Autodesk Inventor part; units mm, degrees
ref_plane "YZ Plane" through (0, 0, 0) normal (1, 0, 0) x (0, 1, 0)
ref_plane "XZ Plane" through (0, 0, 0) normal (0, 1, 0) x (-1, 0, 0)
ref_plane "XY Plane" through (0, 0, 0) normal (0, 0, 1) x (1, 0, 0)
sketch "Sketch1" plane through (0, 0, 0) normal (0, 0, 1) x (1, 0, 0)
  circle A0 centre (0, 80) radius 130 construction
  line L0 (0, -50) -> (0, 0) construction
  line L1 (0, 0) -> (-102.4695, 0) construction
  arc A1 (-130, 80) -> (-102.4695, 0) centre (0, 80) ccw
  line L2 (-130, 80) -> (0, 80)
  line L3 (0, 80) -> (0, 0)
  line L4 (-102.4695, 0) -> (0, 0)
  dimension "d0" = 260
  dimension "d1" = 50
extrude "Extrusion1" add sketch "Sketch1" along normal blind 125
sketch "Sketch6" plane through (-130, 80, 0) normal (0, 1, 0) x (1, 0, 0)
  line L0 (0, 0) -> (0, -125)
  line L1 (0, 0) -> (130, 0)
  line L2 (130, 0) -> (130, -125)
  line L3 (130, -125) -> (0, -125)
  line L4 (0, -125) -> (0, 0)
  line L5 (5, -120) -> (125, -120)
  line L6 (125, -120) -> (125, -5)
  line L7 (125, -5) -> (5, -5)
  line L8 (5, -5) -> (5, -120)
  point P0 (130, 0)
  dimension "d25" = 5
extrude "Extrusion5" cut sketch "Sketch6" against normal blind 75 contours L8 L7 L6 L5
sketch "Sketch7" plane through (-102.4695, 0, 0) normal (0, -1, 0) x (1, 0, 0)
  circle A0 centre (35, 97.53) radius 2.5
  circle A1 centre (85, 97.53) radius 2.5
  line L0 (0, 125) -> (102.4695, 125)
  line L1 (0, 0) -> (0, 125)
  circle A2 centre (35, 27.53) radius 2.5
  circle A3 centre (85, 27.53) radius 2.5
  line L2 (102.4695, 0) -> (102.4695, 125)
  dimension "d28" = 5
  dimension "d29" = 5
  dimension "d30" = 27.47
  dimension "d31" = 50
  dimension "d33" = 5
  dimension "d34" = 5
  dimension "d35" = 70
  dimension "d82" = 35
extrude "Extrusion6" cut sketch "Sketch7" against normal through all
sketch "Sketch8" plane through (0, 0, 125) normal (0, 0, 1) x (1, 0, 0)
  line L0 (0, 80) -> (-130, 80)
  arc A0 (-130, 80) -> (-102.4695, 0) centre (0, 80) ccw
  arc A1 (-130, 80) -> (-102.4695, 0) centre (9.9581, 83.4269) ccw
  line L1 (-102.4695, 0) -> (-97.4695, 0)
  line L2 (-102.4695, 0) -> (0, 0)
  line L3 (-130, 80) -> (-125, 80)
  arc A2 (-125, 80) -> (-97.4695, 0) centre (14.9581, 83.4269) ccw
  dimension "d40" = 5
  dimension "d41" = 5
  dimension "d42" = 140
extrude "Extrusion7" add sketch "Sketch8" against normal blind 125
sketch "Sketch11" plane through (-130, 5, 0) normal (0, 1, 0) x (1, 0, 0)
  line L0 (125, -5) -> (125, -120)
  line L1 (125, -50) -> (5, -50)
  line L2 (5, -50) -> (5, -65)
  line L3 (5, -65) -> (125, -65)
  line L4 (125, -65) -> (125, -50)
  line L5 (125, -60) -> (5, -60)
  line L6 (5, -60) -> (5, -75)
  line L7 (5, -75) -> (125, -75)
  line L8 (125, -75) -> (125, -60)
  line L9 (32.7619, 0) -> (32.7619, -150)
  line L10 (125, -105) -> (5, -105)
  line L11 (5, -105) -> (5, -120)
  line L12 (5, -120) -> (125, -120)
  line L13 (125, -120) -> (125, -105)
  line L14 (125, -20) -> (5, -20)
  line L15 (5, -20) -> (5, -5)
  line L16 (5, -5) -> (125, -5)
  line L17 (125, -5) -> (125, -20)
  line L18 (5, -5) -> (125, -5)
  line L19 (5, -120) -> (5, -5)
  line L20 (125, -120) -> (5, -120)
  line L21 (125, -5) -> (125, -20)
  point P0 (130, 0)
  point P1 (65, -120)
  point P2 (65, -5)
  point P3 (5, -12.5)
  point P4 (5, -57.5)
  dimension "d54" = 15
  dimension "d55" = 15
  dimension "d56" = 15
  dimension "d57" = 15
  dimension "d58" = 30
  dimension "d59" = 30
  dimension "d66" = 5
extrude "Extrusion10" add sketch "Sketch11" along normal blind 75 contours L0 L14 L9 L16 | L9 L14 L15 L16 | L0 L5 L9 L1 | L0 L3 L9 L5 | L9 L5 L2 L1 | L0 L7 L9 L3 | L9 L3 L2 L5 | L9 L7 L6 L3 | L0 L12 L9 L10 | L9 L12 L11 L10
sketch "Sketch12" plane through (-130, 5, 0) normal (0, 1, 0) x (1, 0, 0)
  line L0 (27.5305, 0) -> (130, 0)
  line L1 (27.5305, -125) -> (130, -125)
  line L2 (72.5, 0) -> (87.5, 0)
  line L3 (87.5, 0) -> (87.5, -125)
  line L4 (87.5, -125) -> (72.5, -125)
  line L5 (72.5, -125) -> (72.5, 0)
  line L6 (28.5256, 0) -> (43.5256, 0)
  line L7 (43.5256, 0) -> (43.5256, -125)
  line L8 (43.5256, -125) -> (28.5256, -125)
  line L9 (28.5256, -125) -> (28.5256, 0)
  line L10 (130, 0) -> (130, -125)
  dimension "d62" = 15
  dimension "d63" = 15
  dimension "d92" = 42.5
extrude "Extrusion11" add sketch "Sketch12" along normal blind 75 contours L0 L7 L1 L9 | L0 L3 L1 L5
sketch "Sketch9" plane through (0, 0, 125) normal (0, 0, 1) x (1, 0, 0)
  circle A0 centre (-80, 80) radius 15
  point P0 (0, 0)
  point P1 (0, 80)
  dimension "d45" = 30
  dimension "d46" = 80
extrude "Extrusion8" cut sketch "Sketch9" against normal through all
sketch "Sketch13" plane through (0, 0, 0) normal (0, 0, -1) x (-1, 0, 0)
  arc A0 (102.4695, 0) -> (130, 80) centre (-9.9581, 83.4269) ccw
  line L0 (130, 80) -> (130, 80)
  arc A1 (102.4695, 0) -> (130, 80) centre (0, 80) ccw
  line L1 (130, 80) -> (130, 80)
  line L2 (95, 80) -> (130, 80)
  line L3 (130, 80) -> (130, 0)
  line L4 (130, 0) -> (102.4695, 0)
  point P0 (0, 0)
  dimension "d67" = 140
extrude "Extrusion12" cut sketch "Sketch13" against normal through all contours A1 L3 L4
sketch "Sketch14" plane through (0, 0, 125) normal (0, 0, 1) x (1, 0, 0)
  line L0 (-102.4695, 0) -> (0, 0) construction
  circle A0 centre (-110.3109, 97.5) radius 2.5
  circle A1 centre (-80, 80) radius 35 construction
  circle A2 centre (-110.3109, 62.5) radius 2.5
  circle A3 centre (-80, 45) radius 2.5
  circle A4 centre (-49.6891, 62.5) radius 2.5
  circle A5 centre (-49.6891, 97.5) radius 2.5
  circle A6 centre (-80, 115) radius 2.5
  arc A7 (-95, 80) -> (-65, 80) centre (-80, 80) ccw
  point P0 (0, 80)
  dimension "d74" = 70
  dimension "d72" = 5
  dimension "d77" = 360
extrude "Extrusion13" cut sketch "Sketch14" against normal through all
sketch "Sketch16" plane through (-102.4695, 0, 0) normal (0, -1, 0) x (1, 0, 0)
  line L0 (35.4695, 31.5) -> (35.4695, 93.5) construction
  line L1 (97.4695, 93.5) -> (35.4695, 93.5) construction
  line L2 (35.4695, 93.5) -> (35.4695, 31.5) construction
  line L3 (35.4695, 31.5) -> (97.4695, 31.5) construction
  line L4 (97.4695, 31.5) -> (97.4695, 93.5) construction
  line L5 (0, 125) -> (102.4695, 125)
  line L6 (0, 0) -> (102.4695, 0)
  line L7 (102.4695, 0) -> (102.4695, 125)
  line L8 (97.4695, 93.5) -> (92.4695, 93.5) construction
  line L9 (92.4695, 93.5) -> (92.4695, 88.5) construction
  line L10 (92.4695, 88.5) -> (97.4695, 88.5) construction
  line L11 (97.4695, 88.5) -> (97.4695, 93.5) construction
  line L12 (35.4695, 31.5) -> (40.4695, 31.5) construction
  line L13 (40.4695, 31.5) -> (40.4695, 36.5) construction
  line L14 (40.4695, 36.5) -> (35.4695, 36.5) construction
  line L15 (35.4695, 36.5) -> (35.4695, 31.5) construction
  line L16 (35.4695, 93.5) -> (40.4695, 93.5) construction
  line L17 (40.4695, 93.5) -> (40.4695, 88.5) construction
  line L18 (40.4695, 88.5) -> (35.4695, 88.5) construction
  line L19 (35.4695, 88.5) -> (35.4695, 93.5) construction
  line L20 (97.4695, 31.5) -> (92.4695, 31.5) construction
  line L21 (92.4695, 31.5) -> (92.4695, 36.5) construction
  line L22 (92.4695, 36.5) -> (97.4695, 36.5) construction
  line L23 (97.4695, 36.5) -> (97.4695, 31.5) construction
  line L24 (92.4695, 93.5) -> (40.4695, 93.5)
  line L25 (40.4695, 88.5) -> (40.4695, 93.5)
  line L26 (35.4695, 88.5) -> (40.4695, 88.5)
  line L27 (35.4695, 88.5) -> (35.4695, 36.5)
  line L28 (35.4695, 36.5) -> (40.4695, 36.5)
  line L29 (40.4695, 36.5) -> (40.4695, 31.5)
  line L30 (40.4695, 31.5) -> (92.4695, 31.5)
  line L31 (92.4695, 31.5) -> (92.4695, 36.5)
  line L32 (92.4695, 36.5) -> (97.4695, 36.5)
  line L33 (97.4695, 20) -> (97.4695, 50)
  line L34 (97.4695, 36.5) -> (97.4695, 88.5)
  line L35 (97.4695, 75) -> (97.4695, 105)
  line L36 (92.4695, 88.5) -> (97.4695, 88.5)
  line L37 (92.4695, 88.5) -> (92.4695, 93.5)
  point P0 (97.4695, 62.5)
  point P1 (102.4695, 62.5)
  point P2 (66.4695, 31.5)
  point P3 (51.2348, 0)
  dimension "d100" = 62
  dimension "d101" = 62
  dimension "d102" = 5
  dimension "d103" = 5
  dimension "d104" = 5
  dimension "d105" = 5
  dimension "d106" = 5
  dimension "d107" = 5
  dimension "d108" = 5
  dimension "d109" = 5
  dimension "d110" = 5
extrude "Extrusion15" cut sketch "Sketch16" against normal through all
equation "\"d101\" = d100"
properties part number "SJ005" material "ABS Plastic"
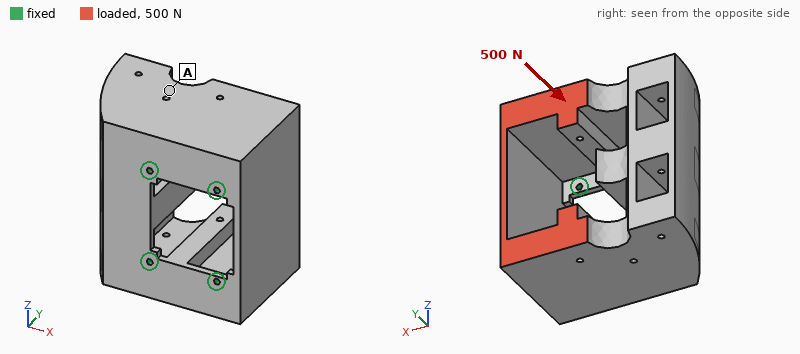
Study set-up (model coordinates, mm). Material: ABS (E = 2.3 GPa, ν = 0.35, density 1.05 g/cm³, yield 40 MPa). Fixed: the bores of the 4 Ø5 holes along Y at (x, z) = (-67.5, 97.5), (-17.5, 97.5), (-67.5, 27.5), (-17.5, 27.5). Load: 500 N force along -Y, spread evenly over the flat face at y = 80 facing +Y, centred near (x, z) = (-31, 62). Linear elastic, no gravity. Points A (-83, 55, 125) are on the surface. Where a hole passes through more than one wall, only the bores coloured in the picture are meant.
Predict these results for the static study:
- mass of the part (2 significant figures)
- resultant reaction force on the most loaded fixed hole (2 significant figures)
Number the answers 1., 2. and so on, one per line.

1. 670 g
2. 180 N
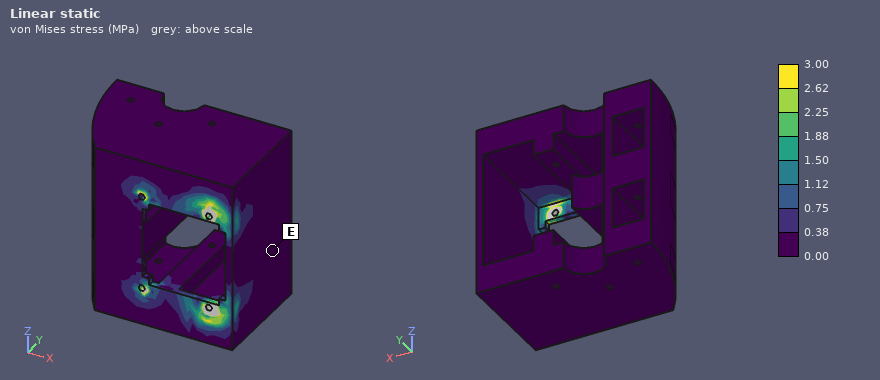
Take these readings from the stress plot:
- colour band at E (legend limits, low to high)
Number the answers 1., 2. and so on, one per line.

1. 0.00 to 0.38 MPa
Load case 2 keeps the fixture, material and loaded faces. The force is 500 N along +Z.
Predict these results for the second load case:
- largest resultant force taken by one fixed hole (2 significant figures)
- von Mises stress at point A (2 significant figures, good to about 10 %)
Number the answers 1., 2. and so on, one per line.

1. 290 N
2. 0.98 MPa
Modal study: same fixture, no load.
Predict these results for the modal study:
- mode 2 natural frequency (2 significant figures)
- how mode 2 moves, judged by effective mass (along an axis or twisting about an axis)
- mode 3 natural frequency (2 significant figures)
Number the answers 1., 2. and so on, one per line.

1. 410 Hz
2. along Z
3. 780 Hz
